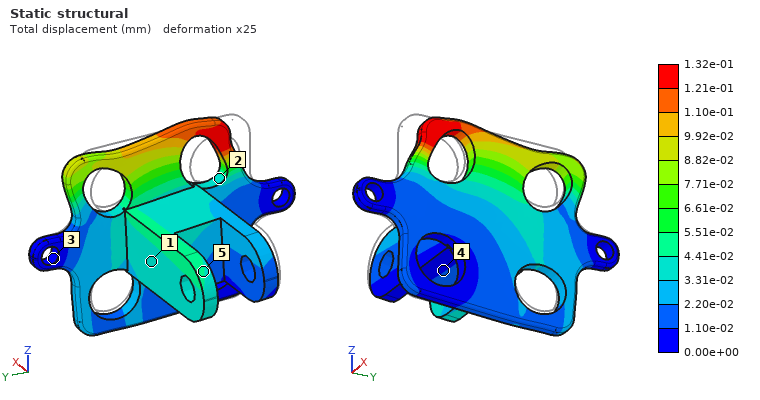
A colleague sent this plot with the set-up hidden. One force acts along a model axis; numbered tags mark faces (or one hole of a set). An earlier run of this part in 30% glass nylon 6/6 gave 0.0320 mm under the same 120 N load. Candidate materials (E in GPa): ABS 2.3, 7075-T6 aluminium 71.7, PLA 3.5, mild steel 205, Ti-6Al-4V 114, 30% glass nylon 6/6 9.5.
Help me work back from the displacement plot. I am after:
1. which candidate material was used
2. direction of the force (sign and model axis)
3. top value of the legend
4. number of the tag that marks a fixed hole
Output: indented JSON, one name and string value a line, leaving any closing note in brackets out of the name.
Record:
{
  "which candidate material was used": "ABS",
  "direction of the force": "+Y",
  "top value of the legend": "1.32e-01 mm",
  "number of the tag that marks a fixed hole": "3"
}
